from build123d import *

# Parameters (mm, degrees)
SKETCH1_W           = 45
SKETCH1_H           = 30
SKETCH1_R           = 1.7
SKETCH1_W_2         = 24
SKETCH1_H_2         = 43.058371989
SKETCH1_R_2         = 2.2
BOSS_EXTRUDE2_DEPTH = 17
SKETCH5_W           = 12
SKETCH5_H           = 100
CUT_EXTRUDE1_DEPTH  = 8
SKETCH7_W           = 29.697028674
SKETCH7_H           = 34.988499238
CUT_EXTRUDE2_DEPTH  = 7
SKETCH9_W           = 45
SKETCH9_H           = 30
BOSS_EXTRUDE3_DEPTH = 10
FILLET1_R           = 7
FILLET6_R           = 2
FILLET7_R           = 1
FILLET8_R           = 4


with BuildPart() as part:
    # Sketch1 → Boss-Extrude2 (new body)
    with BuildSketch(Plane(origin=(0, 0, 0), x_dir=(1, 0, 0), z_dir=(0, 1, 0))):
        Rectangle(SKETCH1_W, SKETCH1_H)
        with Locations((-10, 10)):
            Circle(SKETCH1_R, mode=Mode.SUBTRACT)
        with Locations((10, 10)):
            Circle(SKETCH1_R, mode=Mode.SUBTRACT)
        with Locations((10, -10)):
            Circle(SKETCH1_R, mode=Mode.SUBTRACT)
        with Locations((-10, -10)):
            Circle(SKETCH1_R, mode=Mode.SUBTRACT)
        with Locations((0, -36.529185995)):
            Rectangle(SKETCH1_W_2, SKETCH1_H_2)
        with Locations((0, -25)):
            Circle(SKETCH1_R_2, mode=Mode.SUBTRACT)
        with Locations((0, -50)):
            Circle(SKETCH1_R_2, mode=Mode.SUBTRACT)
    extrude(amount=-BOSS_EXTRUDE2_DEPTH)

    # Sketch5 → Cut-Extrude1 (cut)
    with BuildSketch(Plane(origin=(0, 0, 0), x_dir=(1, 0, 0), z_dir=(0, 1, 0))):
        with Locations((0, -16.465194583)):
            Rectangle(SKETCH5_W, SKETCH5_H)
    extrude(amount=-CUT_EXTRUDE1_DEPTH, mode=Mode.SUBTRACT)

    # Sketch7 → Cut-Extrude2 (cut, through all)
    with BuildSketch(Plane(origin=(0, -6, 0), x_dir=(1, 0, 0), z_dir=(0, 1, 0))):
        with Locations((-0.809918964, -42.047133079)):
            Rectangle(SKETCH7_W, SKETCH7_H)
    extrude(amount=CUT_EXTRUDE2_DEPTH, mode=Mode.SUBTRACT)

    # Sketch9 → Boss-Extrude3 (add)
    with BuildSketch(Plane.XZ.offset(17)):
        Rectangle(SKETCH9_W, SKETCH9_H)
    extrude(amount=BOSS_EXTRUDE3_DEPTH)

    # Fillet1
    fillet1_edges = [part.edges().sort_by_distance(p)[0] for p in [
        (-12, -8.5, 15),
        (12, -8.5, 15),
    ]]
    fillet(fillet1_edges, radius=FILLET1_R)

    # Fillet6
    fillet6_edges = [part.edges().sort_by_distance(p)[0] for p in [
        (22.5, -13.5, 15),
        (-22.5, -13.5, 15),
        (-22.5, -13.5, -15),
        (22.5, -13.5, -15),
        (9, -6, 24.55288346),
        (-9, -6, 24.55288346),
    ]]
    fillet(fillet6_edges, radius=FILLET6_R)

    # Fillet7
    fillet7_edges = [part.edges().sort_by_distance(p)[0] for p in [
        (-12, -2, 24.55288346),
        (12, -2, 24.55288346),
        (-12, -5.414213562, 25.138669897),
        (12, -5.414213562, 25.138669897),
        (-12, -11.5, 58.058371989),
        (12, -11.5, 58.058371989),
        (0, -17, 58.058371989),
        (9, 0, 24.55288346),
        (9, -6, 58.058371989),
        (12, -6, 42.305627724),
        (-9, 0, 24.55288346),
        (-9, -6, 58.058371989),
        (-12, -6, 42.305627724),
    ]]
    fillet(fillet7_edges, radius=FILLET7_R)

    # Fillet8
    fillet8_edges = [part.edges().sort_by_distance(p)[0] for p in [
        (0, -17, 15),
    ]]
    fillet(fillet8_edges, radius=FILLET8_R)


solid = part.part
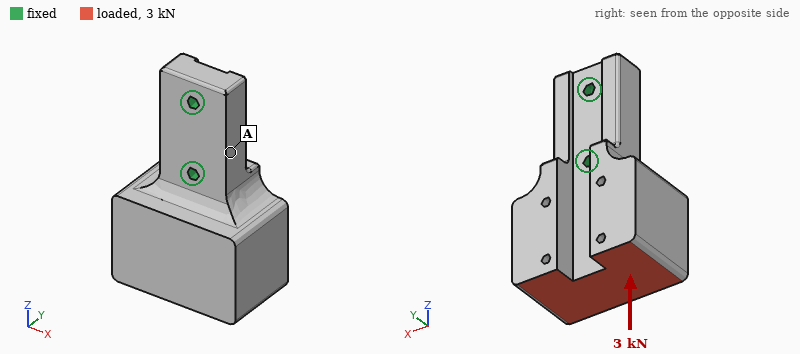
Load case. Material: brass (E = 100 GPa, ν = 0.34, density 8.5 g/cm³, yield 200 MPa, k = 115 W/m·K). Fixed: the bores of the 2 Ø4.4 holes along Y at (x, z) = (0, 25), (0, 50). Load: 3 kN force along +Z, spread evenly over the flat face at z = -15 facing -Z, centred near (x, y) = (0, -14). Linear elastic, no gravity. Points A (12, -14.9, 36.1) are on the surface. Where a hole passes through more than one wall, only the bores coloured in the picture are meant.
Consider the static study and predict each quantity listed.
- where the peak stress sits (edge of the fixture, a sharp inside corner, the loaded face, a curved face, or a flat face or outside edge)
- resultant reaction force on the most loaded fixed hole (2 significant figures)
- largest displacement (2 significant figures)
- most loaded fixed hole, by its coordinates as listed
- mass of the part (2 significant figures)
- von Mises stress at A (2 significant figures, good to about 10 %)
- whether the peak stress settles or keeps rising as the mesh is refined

edge of the fixture
2.5 kN
16 µm
(0, 25)
370 g
5.6 MPa
keeps rising
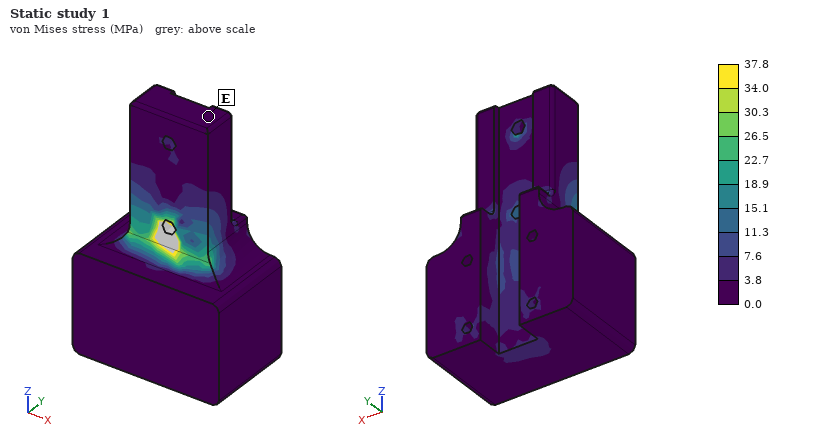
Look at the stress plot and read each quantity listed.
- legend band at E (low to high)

0.0 to 3.8 MPa
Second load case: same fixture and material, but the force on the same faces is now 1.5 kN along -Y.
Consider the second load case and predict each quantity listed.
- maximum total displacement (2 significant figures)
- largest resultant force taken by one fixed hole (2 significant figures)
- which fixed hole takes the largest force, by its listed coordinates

0.11 mm
2.6 kN
(0, 25)
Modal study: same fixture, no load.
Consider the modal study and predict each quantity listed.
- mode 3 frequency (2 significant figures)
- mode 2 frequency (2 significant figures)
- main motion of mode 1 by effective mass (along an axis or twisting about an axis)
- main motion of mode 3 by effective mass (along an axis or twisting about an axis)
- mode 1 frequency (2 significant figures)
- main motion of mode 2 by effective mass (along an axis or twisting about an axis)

2600 Hz
2300 Hz
along Y
twisting about Z
1700 Hz
along X
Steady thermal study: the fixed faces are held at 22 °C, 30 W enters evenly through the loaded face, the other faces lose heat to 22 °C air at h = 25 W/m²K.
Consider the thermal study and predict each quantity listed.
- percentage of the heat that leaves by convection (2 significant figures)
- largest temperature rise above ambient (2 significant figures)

9.2 %
20 K
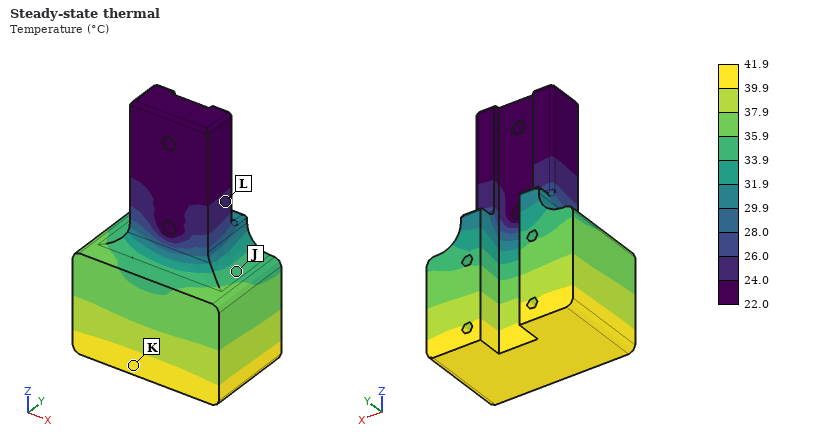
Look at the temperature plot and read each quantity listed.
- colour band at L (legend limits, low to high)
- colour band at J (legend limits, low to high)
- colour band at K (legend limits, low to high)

24.0 to 26.0 °C
33.9 to 35.9 °C
39.9 to 41.9 °C
